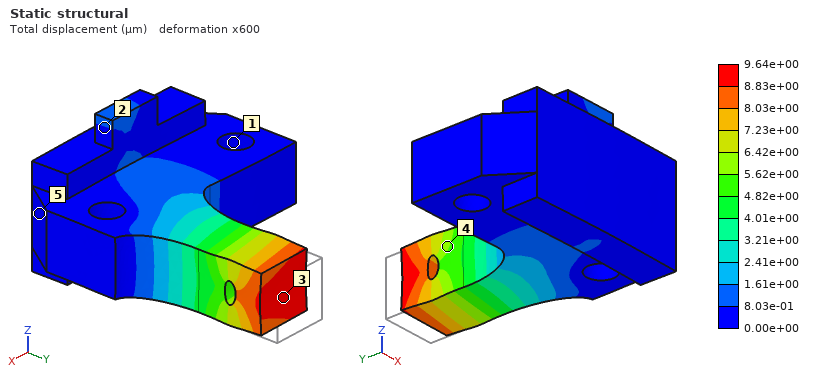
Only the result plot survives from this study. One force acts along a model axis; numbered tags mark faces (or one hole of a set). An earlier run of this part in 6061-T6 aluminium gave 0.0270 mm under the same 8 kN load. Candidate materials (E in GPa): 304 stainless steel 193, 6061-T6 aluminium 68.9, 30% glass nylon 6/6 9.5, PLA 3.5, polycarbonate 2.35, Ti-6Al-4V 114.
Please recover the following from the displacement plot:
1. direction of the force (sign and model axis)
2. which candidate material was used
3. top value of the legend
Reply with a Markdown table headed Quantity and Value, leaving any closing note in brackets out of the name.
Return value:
| Quantity | Value |
|---|---|
| direction of the force | -Y |
| which candidate material was used | 304 stainless steel |
| top value of the legend | 9.64e+00 µm |
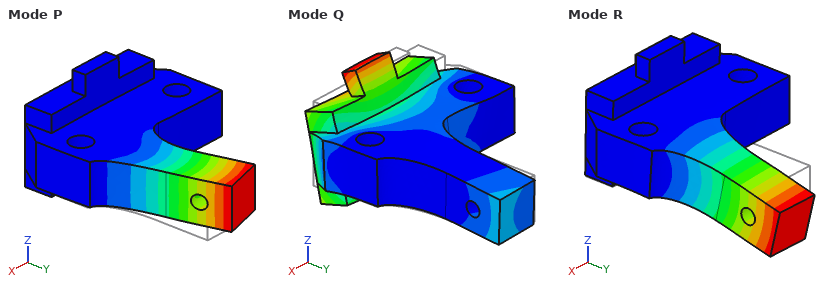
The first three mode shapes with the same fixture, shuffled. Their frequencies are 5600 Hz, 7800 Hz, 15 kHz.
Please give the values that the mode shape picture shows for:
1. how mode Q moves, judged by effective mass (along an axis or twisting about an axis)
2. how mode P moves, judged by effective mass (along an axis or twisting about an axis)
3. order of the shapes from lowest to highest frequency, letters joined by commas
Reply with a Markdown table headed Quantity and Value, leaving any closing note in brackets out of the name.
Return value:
| Quantity | Value |
|---|---|
| how mode Q moves, judged by effective mass | along Z |
| how mode P moves, judged by effective mass | along X |
| order of the shapes from lowest to highest frequency, letters joined by commas | R, P, Q |
